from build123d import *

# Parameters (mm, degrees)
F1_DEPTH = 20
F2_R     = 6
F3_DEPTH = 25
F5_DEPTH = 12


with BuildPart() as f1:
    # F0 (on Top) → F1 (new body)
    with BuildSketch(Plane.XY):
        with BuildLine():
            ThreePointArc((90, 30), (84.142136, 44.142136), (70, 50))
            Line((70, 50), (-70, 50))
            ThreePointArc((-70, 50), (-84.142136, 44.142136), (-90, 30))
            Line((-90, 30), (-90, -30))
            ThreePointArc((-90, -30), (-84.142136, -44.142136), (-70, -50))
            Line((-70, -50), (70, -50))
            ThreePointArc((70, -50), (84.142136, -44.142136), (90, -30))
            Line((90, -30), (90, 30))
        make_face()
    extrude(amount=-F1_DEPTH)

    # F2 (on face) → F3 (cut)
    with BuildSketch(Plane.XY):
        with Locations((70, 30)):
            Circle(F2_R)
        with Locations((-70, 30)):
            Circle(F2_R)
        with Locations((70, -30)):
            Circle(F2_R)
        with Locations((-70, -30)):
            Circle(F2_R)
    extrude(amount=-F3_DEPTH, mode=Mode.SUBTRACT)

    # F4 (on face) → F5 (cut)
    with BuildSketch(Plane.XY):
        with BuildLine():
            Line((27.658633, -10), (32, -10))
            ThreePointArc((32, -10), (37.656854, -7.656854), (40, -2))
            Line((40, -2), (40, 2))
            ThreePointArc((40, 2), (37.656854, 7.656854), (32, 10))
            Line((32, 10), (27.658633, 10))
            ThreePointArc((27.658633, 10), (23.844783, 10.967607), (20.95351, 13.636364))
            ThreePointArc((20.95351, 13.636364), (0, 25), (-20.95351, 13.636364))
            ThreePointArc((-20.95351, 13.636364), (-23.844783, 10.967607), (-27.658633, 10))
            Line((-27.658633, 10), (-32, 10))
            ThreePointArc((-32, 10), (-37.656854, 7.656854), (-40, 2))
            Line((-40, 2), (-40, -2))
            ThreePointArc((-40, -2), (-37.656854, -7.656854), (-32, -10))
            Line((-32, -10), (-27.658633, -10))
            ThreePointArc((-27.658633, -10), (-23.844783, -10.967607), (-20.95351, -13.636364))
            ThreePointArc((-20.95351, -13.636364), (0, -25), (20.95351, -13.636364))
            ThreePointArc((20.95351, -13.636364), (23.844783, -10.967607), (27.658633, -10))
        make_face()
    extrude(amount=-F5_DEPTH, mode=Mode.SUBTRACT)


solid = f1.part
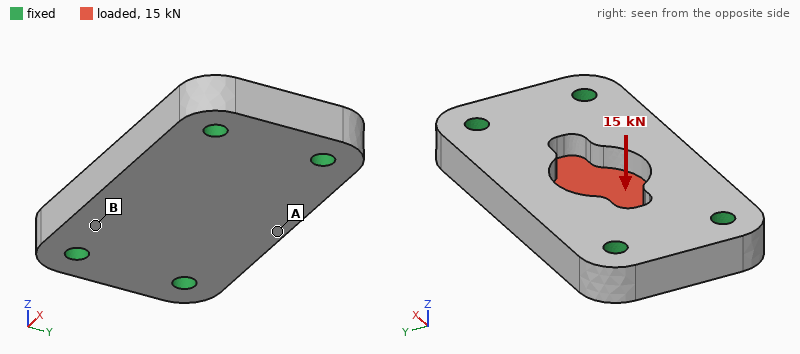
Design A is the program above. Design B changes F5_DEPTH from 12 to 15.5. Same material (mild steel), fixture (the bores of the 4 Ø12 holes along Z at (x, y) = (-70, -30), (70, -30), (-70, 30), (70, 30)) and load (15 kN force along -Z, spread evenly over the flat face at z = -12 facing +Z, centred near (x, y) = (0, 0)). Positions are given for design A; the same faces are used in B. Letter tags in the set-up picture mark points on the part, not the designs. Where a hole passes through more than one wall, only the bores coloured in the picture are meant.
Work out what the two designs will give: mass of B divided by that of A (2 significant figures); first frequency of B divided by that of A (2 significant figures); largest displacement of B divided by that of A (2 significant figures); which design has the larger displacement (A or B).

0.97
1.0
1.9
B
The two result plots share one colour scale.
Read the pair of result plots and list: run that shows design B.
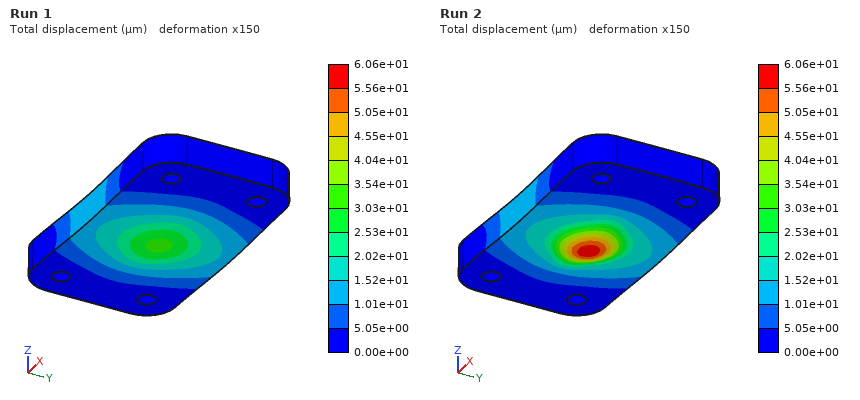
Run 2
